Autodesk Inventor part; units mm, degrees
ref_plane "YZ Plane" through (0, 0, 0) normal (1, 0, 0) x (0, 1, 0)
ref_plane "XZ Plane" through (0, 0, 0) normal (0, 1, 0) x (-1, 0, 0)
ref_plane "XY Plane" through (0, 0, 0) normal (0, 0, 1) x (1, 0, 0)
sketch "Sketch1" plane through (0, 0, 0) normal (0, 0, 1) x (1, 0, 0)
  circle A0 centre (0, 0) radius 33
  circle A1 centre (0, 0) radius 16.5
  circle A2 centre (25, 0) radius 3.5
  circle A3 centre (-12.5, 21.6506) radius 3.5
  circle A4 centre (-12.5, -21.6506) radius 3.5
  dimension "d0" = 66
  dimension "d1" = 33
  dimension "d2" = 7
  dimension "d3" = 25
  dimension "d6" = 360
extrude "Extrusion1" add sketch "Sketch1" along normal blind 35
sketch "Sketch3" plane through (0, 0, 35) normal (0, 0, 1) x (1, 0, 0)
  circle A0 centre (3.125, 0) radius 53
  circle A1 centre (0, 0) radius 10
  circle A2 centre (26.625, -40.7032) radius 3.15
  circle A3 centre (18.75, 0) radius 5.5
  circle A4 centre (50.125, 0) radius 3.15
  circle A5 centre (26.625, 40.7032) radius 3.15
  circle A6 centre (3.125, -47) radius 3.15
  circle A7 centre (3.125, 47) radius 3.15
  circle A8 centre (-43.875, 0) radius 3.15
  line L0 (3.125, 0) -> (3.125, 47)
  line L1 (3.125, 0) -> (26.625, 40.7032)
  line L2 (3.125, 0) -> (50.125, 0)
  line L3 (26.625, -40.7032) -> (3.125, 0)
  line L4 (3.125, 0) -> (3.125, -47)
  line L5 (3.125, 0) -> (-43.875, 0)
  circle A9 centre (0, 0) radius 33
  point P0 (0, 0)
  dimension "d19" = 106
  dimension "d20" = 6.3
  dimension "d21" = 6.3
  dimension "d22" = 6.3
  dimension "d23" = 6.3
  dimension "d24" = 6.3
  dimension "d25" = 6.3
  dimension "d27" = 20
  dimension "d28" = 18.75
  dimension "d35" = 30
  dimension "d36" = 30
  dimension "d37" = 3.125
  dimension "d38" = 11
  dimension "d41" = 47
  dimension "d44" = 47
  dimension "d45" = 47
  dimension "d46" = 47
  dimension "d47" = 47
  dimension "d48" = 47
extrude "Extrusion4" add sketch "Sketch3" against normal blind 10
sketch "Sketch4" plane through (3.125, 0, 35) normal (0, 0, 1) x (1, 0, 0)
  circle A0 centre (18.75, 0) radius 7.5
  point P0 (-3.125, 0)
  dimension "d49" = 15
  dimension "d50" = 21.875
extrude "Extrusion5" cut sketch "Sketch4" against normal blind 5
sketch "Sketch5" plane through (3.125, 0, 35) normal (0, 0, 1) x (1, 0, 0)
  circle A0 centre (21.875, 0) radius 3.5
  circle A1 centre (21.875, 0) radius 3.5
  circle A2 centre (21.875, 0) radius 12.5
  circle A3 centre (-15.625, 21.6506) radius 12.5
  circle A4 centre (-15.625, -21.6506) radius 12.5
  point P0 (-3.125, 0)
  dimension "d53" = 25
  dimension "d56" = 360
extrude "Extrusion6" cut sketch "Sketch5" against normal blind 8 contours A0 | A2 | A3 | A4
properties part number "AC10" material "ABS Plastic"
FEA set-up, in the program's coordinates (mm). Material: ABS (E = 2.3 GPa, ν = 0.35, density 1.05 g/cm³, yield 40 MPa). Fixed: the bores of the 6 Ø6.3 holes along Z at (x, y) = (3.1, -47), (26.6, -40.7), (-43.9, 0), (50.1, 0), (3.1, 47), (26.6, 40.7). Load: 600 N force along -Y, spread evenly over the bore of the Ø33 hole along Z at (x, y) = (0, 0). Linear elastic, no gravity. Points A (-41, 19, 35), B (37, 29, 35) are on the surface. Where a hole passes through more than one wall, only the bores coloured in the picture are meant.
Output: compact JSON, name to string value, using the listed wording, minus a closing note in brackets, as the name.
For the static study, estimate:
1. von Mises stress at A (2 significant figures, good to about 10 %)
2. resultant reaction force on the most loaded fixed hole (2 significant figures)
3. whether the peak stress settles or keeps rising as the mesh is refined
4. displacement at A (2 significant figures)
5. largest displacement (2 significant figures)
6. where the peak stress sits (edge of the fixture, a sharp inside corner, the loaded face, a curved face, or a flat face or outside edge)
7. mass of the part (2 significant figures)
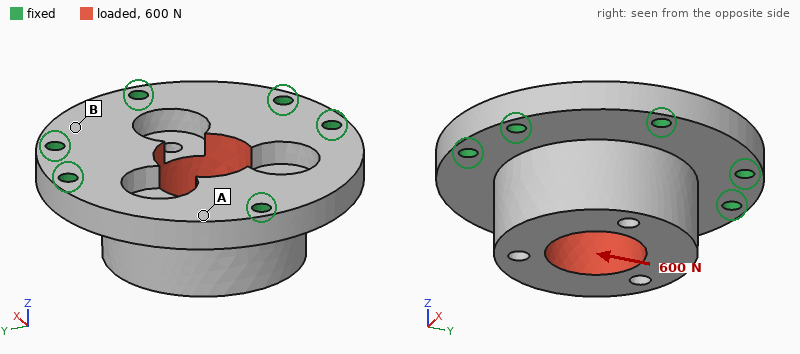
{"von Mises stress at A": "0.36 MPa", "resultant reaction force on the most loaded fixed hole": "150 N", "whether the peak stress settles or keeps rising as the mesh is refined": "keeps rising", "displacement at A": "7.0 µm", "largest displacement": "26 µm", "where the peak stress sits": "edge of the fixture", "mass of the part": "130 g"}
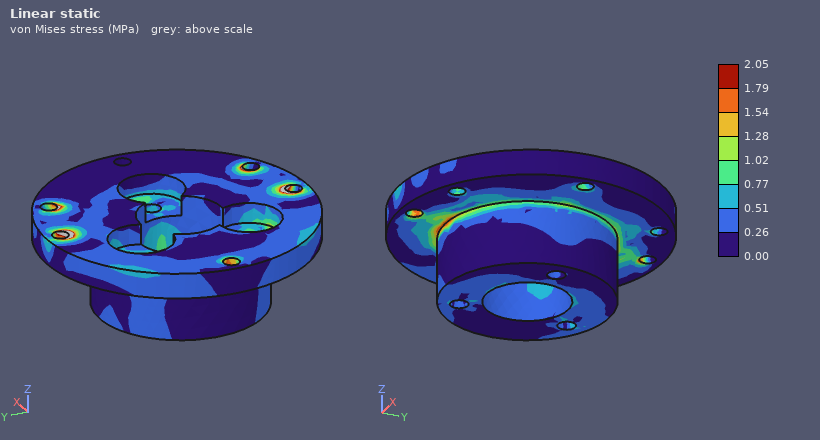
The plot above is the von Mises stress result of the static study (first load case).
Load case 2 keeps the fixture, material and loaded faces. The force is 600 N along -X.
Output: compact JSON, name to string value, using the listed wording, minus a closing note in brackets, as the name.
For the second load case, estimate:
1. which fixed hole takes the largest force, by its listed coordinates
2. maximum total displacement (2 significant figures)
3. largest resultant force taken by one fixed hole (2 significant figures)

{"which fixed hole takes the largest force, by its listed coordinates": "(-43.9, 0)", "maximum total displacement": "28 µm", "largest resultant force taken by one fixed hole": "210 N"}
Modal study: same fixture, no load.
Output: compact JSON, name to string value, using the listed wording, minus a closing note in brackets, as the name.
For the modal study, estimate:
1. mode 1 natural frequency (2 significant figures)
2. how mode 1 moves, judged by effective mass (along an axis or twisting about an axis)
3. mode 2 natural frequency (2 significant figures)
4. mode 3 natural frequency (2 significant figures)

{"mode 1 natural frequency": "2400 Hz", "how mode 1 moves, judged by effective mass": "along Z", "mode 2 natural frequency": "2600 Hz", "mode 3 natural frequency": "2700 Hz"}
